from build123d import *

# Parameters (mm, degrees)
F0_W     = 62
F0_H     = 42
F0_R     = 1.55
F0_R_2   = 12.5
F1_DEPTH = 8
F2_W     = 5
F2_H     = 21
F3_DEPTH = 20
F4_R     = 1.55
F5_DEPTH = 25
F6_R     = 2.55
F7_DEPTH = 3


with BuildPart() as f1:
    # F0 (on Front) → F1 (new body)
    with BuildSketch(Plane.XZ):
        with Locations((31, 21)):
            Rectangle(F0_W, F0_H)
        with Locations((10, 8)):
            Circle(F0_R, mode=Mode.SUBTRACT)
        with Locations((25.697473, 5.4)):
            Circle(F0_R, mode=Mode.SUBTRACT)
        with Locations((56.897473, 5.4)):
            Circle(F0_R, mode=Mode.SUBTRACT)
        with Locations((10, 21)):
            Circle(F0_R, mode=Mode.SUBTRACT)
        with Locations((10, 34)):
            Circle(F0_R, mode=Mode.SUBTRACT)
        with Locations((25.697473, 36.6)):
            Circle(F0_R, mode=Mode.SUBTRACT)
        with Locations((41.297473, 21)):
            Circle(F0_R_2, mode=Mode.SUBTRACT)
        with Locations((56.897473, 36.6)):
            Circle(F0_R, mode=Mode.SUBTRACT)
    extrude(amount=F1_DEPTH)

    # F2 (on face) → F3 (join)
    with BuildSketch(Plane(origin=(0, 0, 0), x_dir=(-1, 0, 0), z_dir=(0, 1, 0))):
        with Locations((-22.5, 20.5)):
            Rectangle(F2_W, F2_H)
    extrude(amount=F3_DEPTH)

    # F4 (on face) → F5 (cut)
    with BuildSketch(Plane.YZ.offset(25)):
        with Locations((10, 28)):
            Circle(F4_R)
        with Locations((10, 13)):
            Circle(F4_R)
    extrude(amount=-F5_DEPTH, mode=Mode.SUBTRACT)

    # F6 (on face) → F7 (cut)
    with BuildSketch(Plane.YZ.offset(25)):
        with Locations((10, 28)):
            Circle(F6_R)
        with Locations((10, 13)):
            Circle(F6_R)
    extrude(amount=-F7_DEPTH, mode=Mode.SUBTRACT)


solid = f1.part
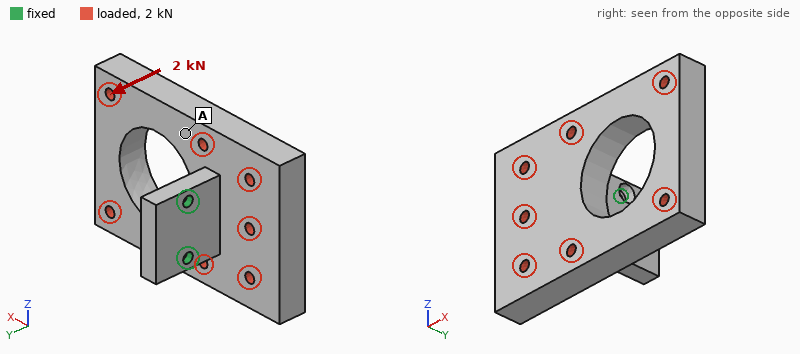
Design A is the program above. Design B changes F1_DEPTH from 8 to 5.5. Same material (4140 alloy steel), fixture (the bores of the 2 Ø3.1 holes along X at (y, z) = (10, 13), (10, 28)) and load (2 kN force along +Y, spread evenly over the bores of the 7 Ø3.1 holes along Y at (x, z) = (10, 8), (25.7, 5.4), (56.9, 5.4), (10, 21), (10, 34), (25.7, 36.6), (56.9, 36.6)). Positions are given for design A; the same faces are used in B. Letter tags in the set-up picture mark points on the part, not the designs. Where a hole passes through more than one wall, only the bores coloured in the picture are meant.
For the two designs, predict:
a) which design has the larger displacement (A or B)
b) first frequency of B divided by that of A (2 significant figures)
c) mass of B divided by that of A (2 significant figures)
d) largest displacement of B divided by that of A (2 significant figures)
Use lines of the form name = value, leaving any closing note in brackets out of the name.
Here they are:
which design has the larger displacement = B
first frequency of B divided by that of A = 1.2
mass of B divided by that of A = 0.72
largest displacement of B divided by that of A = 1.3
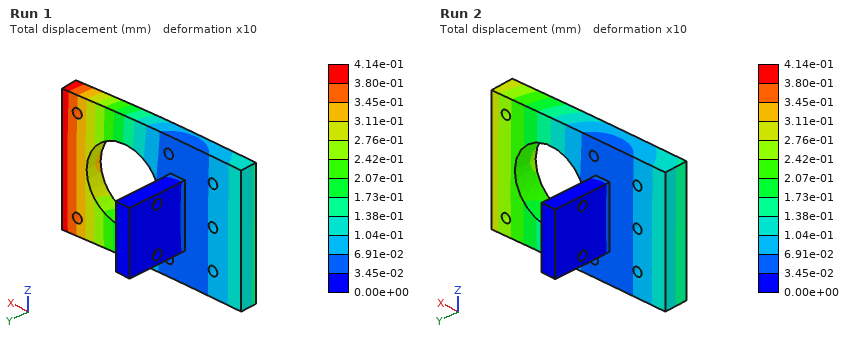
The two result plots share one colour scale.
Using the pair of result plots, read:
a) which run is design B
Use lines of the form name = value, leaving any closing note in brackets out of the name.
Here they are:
which run is design B = Run 1
